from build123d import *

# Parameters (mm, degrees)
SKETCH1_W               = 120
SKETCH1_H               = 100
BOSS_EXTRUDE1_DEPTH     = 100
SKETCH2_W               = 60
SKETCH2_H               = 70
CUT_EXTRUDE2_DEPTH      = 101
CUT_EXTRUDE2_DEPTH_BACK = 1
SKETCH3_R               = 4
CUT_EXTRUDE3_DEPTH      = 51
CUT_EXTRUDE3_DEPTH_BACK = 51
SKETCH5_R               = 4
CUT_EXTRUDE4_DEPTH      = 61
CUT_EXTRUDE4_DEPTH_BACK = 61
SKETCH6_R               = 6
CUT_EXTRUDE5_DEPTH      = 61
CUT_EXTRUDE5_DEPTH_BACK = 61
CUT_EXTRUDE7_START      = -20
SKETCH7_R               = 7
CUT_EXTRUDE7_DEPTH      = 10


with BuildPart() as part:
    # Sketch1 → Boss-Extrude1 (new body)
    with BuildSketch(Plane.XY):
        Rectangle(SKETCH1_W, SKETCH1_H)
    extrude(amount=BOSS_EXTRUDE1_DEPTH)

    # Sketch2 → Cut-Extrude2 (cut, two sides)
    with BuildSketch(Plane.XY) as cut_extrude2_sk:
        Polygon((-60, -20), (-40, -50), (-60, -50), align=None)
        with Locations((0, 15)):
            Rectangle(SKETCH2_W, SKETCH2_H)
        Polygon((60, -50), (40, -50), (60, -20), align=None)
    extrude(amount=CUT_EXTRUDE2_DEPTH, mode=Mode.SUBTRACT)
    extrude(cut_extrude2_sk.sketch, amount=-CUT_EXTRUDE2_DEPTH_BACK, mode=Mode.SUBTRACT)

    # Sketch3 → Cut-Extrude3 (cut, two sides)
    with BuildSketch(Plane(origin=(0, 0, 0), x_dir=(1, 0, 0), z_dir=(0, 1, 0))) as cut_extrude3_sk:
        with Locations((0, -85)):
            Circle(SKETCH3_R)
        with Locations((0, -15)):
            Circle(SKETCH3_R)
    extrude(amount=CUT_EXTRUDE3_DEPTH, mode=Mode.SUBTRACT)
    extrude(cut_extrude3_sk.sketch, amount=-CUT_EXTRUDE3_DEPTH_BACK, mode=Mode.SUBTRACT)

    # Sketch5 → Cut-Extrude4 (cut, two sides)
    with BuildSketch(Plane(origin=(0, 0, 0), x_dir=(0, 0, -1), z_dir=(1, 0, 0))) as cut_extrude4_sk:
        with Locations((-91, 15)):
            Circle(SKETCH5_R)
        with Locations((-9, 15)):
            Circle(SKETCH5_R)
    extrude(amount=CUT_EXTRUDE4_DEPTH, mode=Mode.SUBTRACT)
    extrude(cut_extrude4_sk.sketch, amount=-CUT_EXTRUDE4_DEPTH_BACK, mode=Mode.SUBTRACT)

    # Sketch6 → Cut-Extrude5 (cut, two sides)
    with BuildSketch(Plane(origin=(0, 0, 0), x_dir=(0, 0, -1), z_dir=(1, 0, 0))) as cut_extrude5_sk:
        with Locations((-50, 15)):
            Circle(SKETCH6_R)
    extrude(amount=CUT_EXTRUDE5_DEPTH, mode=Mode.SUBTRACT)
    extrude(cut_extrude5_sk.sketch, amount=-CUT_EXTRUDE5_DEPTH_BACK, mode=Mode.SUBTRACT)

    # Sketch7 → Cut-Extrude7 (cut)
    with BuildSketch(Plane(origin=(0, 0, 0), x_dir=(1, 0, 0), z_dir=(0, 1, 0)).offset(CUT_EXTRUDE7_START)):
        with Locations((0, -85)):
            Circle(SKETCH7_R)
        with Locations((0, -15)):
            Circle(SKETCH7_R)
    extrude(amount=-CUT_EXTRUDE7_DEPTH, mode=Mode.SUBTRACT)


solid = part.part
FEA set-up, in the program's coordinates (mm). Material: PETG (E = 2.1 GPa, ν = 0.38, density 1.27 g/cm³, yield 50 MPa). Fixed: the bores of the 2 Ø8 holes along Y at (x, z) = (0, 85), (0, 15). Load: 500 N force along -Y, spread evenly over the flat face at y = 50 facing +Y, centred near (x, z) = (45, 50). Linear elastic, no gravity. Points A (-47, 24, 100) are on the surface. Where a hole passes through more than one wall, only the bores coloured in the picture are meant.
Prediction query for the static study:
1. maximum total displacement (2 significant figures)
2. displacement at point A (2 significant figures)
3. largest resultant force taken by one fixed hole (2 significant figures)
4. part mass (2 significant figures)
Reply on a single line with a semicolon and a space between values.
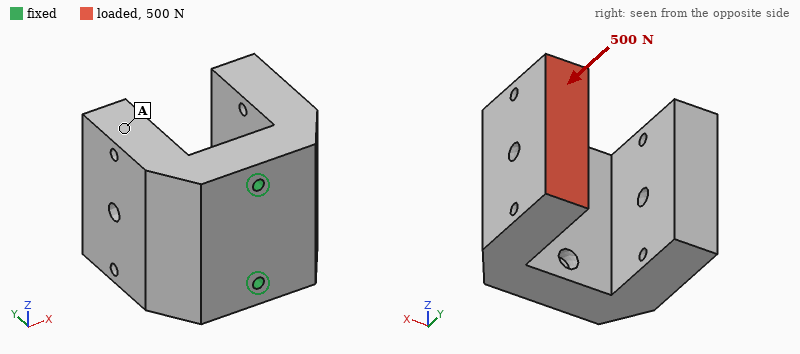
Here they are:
0.29 mm; 0.12 mm; 250 N; 890 g
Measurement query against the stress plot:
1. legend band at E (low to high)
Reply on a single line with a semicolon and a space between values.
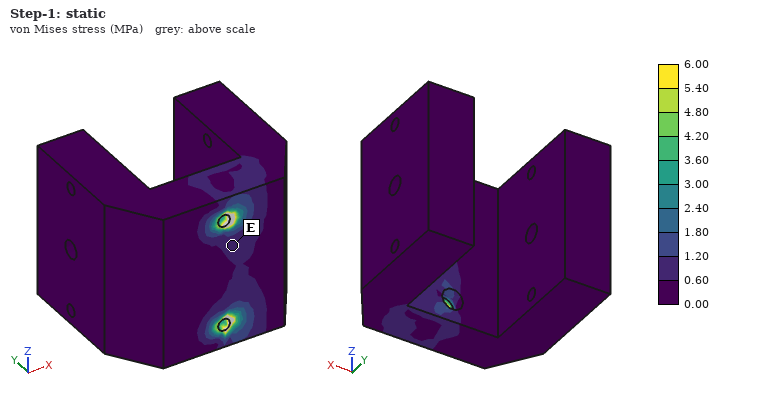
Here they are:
0.60 to 1.20 MPa
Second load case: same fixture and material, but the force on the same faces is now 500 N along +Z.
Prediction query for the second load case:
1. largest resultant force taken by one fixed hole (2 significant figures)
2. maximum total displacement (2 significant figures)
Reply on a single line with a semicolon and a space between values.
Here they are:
710 N; 0.25 mm
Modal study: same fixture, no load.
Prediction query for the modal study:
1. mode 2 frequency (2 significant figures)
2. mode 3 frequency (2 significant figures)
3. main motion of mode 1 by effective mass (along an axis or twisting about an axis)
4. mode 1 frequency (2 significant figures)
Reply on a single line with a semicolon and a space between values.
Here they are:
460 Hz; 670 Hz; along X; 280 Hz
